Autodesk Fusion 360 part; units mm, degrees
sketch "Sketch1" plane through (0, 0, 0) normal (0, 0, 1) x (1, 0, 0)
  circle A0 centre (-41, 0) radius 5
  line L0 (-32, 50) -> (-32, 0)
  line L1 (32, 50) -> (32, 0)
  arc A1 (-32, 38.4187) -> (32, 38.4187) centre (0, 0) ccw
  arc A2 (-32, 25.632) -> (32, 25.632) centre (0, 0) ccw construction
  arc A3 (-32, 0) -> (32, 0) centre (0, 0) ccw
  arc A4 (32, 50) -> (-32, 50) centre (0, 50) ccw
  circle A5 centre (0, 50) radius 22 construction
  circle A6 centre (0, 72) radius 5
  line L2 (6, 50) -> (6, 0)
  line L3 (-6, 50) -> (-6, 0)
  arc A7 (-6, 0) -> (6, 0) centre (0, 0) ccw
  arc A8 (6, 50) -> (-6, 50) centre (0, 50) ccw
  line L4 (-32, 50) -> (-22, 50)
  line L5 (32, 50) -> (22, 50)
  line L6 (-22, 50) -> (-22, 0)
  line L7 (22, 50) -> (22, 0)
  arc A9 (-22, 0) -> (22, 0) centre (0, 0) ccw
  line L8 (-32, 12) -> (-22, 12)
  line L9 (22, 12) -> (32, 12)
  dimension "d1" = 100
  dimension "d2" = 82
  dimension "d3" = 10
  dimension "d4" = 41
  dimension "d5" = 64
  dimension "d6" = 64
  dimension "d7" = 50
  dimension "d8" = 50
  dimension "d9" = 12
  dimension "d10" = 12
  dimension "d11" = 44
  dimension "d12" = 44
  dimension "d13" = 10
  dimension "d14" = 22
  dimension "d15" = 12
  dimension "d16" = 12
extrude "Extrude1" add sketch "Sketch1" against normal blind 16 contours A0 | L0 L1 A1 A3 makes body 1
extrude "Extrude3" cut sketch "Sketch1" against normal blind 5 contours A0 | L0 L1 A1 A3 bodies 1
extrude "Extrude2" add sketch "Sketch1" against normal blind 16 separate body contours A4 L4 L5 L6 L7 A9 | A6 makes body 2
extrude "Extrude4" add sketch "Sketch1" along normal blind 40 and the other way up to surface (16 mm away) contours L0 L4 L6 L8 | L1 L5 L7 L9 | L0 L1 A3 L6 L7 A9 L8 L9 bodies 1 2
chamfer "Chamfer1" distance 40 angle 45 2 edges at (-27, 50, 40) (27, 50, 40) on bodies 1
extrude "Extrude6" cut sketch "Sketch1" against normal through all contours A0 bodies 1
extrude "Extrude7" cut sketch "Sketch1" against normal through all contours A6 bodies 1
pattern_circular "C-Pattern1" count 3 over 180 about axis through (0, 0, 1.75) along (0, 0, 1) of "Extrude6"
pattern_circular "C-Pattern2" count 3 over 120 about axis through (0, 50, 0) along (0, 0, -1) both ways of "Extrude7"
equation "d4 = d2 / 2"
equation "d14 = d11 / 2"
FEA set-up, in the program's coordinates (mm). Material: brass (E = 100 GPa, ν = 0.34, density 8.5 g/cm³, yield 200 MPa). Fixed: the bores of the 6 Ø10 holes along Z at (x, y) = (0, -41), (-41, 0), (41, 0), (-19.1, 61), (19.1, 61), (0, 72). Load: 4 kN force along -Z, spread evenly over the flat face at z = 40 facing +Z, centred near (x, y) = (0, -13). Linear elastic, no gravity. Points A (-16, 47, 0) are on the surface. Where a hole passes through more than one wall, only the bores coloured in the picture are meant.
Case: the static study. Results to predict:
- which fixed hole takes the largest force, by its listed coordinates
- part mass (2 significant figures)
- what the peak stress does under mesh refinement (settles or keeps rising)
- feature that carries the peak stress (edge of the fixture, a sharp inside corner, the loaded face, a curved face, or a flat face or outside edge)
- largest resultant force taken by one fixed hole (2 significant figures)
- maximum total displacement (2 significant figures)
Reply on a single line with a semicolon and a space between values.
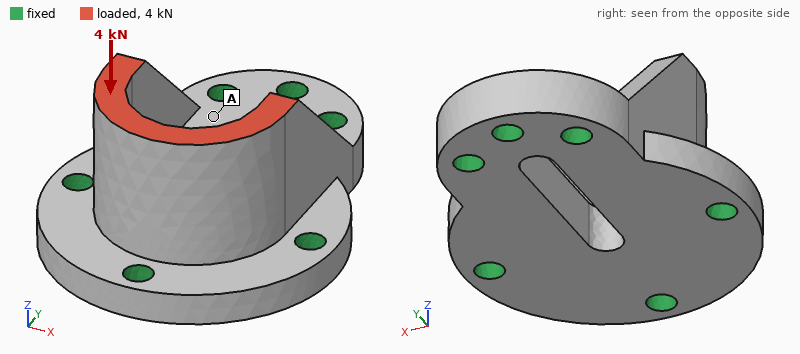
(0, -41); 1.5 kg; keeps rising; edge of the fixture; 1.7 kN; 5.0 µm
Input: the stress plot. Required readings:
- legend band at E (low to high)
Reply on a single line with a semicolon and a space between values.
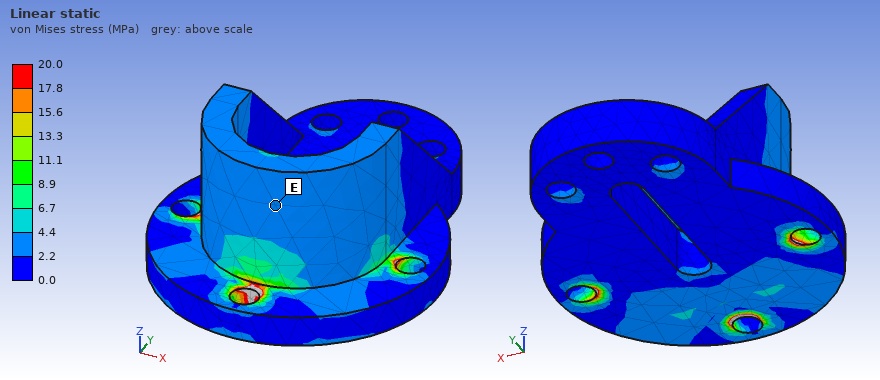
2.2 to 4.4 MPa
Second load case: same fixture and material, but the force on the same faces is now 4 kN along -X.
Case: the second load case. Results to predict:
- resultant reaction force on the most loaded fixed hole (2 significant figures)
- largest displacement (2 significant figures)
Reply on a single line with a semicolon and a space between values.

3.3 kN; 38 µm
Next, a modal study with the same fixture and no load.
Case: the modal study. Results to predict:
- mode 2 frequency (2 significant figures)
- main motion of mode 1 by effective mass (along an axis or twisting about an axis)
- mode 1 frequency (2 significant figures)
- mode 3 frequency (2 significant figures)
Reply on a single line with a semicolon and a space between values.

5000 Hz; along X; 4400 Hz; 6600 Hz
